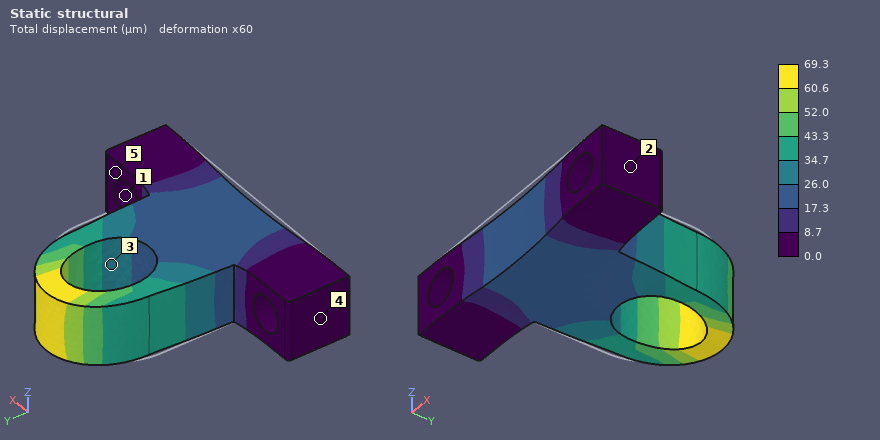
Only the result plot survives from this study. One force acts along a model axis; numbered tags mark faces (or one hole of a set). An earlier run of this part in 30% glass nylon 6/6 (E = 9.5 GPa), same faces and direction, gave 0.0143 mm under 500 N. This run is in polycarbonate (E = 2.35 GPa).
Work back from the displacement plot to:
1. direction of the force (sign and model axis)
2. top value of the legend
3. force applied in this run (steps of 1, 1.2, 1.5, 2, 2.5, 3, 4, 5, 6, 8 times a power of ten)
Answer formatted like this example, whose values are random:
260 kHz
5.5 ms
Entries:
+Y
69.3 µm
600 N
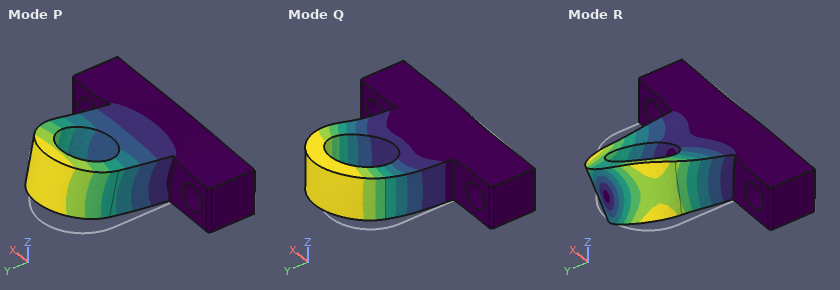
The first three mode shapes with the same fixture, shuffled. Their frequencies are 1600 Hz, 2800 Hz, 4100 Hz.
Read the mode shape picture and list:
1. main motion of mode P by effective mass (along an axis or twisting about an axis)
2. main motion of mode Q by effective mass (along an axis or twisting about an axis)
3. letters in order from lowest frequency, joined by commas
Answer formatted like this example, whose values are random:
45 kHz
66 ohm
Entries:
along Z
along X
P, Q, R
